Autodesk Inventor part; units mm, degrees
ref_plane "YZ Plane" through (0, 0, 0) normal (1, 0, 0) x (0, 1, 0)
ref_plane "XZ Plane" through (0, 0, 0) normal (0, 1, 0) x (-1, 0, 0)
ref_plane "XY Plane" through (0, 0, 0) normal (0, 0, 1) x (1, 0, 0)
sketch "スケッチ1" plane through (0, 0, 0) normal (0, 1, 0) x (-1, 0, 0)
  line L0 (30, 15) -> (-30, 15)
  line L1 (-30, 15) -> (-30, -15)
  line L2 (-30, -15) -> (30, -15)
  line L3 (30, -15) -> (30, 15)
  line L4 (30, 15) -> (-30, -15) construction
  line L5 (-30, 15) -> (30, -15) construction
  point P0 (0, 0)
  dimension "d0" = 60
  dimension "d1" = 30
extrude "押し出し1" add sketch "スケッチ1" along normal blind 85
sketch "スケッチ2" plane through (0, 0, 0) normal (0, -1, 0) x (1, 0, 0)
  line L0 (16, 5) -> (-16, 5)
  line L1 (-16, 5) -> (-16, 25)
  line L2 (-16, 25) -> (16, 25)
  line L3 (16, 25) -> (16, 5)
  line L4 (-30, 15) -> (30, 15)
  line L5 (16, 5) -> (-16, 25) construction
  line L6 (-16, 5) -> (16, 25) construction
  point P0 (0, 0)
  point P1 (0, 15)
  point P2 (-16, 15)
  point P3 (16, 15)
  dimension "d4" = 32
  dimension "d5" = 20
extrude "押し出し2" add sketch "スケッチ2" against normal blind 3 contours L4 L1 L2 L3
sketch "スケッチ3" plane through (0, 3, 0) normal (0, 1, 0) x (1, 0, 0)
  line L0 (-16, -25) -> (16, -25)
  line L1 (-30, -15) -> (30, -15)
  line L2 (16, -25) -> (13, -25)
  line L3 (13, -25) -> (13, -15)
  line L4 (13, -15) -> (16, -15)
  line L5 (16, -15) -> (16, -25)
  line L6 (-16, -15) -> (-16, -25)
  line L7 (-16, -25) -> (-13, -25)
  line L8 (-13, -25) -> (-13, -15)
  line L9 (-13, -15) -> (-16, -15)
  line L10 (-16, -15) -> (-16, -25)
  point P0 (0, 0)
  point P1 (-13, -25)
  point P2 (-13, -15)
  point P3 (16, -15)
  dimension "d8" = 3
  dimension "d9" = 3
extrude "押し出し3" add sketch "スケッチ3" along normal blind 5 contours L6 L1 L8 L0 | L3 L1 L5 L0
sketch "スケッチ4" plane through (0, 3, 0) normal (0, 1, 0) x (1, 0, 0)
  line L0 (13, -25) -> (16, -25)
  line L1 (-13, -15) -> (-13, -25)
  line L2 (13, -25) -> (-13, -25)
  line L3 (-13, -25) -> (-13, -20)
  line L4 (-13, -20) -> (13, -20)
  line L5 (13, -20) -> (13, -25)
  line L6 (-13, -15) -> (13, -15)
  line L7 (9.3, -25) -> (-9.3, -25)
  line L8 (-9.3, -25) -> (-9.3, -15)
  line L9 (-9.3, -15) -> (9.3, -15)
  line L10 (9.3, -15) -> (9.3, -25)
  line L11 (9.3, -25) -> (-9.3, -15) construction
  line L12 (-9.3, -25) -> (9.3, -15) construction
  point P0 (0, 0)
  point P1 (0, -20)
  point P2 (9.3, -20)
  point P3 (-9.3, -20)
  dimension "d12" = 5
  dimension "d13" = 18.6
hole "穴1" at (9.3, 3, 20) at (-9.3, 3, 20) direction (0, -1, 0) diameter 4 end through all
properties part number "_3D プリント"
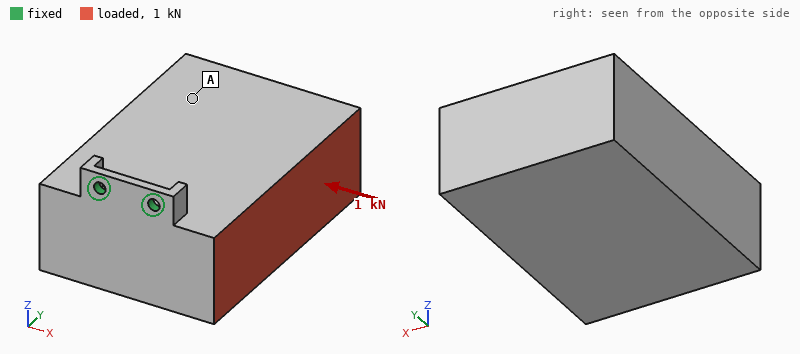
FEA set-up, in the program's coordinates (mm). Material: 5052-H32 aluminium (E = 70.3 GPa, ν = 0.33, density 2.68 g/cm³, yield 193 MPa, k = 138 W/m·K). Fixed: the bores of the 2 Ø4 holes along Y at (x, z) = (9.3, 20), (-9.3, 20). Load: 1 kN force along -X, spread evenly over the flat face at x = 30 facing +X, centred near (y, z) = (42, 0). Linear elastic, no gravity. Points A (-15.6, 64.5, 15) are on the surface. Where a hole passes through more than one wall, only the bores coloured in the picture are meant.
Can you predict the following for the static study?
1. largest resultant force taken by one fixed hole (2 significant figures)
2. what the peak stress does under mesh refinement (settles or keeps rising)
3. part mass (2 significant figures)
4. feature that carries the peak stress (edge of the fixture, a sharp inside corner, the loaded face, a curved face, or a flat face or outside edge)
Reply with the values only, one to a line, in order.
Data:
2.1 kN
keeps rising
410 g
edge of the fixture
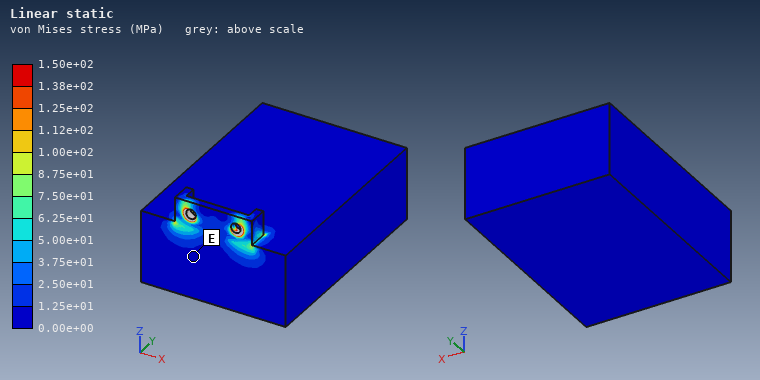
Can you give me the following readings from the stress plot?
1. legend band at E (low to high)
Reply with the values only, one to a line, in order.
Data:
0.00e+00 to 1.25e+01 MPa
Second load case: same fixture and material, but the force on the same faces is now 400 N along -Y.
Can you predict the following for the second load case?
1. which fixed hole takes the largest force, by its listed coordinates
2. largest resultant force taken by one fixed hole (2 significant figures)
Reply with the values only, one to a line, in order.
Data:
(9.3, 20)
730 N
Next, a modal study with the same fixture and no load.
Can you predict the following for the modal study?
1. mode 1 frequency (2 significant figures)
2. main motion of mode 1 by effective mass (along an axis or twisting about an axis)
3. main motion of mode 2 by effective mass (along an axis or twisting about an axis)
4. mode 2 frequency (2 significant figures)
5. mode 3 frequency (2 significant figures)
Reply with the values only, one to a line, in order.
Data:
200 Hz
along Z
along X
640 Hz
2300 Hz
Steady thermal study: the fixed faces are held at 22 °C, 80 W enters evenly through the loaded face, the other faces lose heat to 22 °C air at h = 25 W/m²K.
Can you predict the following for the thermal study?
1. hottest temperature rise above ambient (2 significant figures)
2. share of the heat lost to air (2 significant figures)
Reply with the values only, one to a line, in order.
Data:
51 K
22 %
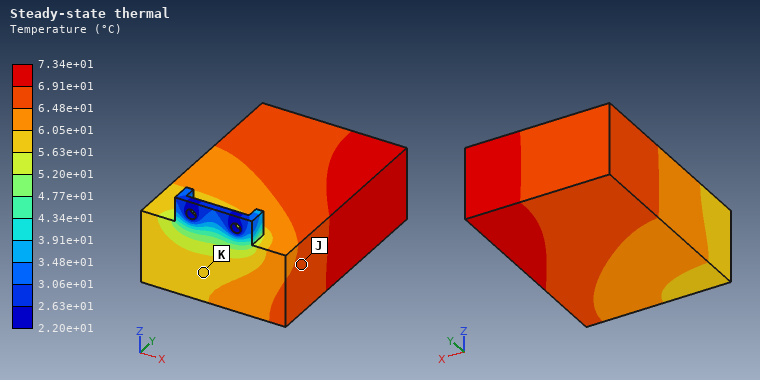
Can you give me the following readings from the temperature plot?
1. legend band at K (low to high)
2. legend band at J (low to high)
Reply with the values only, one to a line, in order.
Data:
5.63e+01 to 6.05e+01 °C
6.48e+01 to 6.91e+01 °C
